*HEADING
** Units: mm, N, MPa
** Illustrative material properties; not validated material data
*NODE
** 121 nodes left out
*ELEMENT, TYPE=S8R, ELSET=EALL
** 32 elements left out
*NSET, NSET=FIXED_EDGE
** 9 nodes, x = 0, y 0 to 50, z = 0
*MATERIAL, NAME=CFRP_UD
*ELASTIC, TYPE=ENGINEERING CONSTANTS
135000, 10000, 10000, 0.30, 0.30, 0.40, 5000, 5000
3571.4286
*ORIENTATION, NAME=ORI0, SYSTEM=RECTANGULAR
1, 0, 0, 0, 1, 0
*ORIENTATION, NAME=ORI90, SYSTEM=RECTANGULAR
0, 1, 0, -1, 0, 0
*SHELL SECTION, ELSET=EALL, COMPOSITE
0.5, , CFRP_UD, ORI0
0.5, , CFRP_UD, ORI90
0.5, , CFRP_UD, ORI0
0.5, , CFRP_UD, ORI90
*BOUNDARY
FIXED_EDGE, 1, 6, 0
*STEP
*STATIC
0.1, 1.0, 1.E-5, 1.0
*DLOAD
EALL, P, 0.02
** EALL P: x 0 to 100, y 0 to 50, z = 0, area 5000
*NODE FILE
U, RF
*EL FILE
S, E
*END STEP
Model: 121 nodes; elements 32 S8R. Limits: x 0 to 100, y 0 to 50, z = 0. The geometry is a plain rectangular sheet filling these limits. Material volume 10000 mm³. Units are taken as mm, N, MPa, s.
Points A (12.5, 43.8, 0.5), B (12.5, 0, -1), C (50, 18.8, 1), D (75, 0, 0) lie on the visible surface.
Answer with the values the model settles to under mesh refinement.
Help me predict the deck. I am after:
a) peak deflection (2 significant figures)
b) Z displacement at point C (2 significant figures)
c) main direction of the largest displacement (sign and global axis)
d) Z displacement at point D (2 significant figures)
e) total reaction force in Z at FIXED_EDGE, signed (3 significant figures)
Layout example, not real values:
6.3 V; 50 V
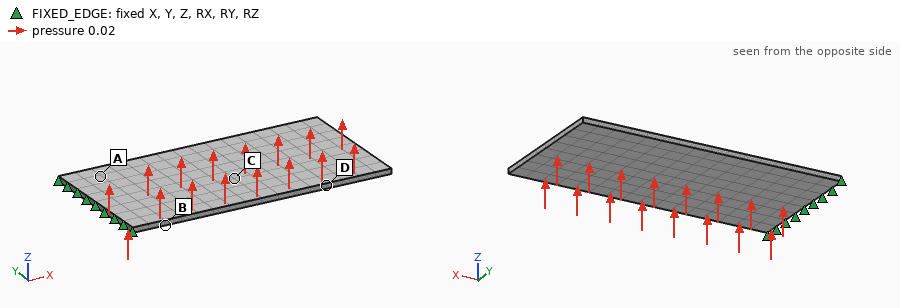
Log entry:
6.0 mm; 2.1 mm; +Z; 4.0 mm; -100 N
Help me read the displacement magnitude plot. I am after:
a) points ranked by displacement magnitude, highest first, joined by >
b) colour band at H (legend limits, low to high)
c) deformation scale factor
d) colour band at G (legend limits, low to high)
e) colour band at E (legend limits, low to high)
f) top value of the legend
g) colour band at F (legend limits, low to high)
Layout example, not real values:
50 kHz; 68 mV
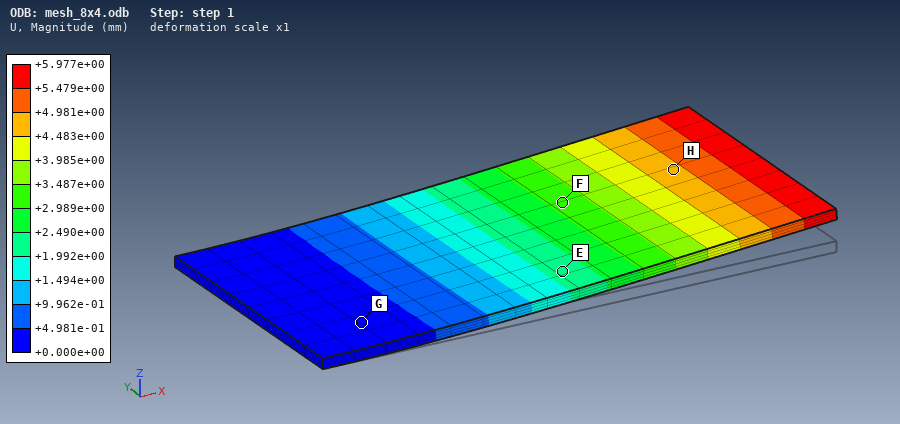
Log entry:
H > F > E > G; +4.483e+00 to +4.981e+00 mm; 1; +0.000e+00 to +4.981e-01 mm; +1.992e+00 to +2.490e+00 mm; +5.977e+00 mm; +2.989e+00 to +3.487e+00 mm
